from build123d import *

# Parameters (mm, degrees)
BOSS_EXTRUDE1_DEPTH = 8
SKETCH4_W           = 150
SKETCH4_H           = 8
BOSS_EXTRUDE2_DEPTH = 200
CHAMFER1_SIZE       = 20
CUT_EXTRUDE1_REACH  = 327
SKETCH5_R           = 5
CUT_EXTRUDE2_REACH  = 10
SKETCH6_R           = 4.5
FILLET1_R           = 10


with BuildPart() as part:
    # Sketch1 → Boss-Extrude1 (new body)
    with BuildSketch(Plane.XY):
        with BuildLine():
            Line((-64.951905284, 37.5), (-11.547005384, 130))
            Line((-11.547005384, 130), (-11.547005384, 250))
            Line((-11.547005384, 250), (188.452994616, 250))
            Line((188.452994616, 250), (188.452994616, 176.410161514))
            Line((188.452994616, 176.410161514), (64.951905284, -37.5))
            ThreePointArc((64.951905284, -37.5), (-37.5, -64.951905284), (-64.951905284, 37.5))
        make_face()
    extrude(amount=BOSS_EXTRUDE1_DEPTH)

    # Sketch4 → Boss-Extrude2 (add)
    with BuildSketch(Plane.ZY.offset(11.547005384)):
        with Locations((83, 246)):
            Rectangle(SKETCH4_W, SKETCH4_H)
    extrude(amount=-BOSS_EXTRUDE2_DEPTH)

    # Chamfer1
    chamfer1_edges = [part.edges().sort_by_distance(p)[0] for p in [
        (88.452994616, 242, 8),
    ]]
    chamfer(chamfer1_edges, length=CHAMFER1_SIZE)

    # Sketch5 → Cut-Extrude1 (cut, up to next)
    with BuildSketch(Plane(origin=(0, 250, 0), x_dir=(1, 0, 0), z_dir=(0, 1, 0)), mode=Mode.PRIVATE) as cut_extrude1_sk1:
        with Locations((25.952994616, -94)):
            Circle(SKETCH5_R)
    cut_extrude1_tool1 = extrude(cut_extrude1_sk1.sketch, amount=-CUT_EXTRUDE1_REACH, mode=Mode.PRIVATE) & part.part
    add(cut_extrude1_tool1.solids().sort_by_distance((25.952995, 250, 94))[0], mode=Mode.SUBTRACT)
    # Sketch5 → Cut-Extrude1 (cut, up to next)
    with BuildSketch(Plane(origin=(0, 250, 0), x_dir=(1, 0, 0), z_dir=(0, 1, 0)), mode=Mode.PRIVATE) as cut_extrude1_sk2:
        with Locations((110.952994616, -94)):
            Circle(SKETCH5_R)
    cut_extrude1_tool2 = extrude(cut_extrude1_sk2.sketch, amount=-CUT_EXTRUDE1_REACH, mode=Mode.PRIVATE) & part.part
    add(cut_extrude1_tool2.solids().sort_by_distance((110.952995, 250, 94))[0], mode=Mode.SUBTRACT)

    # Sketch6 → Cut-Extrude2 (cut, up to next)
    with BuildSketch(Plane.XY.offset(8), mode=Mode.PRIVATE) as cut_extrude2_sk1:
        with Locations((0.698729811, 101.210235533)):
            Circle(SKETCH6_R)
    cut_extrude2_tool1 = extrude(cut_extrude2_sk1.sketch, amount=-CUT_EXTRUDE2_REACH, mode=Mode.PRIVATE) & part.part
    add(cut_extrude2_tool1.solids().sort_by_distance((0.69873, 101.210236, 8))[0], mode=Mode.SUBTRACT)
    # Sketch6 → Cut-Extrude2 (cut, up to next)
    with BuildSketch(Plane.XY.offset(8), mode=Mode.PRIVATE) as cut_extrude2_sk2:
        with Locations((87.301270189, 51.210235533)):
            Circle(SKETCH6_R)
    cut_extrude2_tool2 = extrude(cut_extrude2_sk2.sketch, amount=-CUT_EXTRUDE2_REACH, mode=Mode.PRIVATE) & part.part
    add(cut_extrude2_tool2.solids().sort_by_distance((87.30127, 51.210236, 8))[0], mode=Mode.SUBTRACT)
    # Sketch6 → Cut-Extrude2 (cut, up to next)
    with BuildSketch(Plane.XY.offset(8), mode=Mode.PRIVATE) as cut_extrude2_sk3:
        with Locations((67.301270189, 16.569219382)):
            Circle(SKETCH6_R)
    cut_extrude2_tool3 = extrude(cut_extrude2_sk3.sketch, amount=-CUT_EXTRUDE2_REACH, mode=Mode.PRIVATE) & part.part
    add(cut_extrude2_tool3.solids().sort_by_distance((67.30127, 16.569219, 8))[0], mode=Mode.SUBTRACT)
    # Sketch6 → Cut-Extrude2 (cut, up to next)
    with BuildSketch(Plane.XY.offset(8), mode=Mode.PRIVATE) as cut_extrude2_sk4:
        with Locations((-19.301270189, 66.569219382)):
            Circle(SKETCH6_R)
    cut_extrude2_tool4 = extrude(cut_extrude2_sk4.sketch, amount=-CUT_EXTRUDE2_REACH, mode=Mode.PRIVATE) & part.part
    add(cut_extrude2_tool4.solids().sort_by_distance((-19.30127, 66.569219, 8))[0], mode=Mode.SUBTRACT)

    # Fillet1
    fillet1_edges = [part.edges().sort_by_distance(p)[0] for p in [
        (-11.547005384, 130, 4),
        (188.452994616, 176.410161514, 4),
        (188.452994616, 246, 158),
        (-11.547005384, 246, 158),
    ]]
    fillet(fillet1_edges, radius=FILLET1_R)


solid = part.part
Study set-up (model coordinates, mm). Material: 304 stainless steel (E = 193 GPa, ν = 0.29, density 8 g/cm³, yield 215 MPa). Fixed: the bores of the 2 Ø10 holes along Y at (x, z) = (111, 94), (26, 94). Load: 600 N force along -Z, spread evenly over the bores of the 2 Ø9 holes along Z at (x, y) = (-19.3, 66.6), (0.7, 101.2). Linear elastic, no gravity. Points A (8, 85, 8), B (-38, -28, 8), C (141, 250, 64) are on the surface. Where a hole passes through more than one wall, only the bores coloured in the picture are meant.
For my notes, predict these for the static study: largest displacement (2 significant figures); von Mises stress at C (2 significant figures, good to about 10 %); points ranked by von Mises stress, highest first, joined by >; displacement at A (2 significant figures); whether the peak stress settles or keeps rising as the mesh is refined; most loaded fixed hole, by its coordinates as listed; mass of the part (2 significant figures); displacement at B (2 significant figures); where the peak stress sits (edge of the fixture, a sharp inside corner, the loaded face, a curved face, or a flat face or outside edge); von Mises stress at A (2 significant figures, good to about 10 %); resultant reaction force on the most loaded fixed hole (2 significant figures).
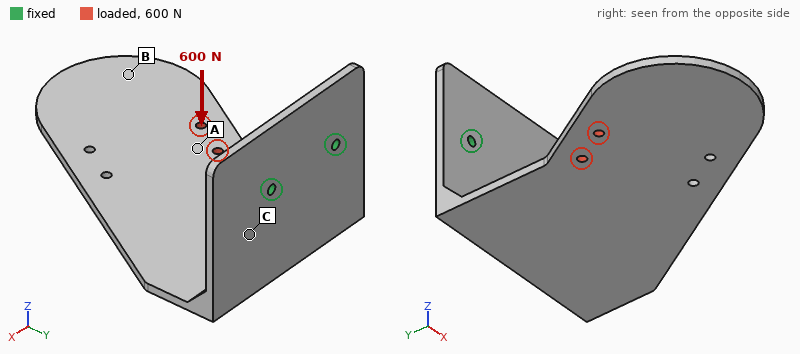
2.7 mm
37 MPa
C > A > B
1.3 mm
keeps rising
(26, 94)
5.7 kg
2.4 mm
edge of the fixture
13 MPa
820 N
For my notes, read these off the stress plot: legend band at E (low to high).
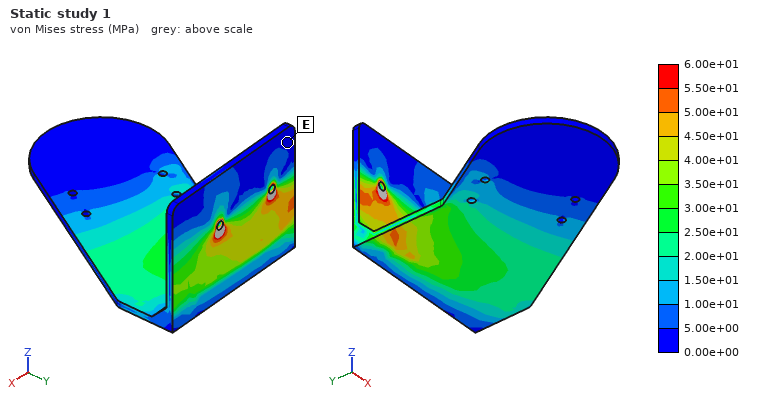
0.00e+00 to 5.00e+00 MPa
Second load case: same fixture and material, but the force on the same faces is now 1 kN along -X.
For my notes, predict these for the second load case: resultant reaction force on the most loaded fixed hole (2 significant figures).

1.9 kN
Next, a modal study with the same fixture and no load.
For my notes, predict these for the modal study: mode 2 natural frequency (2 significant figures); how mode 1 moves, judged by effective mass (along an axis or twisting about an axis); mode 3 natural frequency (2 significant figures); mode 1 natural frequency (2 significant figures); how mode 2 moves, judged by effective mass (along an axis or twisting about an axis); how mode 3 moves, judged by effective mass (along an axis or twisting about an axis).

140 Hz
along Z
210 Hz
54 Hz
along X
along Y
